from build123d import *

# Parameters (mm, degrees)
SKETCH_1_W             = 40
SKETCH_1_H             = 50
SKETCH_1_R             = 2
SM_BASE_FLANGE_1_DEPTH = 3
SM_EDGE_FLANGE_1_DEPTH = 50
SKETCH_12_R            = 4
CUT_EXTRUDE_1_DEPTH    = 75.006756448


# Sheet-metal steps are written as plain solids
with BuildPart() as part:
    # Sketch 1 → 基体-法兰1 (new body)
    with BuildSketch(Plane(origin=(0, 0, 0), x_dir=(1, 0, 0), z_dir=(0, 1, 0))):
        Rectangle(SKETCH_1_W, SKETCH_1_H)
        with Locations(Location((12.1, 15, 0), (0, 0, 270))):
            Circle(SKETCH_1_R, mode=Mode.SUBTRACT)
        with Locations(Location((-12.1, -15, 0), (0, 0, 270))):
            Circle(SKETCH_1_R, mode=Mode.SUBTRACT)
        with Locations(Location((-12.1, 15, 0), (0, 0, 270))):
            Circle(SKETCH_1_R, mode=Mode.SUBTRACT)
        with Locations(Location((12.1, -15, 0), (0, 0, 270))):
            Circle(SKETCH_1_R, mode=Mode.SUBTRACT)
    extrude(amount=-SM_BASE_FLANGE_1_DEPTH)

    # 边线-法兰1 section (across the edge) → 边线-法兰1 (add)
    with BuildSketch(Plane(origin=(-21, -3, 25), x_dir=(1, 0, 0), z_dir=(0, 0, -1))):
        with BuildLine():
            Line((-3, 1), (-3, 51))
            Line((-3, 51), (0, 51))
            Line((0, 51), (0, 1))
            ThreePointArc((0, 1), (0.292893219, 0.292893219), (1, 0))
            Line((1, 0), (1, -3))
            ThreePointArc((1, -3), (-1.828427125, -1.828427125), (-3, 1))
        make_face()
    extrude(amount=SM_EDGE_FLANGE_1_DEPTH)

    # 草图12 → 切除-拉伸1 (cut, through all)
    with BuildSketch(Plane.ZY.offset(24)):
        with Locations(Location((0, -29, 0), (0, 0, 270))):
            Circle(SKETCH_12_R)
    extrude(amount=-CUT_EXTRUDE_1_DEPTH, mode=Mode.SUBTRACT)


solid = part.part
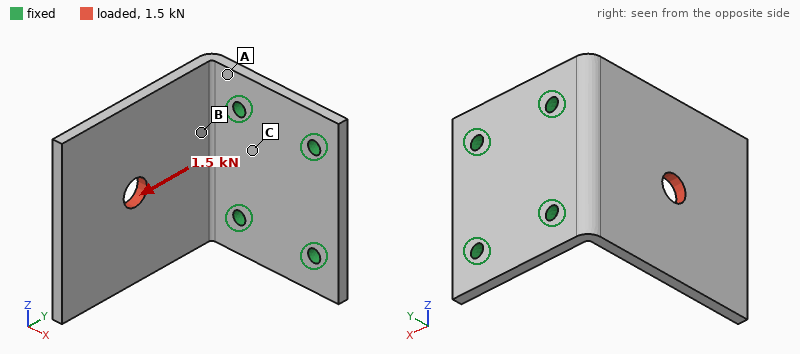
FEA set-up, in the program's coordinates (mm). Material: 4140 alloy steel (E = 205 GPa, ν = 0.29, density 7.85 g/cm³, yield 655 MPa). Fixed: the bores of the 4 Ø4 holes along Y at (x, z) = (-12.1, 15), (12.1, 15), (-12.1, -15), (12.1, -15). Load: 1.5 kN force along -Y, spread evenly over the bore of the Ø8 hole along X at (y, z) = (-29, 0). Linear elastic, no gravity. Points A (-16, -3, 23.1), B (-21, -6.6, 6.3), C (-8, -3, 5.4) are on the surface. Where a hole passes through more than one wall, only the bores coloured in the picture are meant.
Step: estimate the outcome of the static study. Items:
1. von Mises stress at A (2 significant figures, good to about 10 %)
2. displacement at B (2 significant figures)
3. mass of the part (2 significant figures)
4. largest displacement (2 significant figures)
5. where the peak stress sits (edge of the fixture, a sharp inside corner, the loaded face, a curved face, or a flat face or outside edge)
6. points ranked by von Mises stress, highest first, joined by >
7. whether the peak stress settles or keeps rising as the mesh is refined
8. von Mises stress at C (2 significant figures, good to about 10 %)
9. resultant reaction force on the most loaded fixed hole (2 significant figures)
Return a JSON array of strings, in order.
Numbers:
["100 MPa", "0.029 mm", "110 g", "0.19 mm", "edge of the fixture", "A > C > B", "keeps rising", "43 MPa", "820 N"]
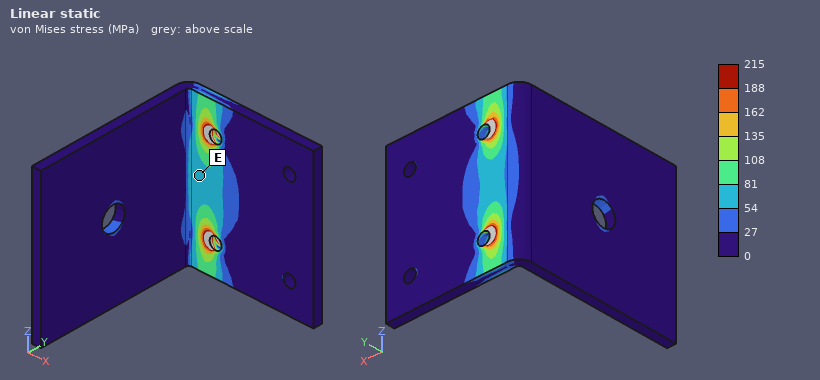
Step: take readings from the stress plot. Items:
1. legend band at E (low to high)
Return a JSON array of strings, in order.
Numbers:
["54 to 81 MPa"]
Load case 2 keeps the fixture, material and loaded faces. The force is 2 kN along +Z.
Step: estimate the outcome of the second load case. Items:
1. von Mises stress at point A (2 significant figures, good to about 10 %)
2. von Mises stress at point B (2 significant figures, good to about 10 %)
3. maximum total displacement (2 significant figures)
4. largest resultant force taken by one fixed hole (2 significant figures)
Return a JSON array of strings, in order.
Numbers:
["160 MPa", "120 MPa", "0.19 mm", "2.1 kN"]
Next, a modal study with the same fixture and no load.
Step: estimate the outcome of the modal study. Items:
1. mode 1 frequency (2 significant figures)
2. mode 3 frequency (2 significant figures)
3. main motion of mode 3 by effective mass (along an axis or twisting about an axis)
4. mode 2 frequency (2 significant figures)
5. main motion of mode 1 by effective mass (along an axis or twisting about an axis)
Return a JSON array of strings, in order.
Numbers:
["700 Hz", "3000 Hz", "along Z", "1900 Hz", "along X"]
